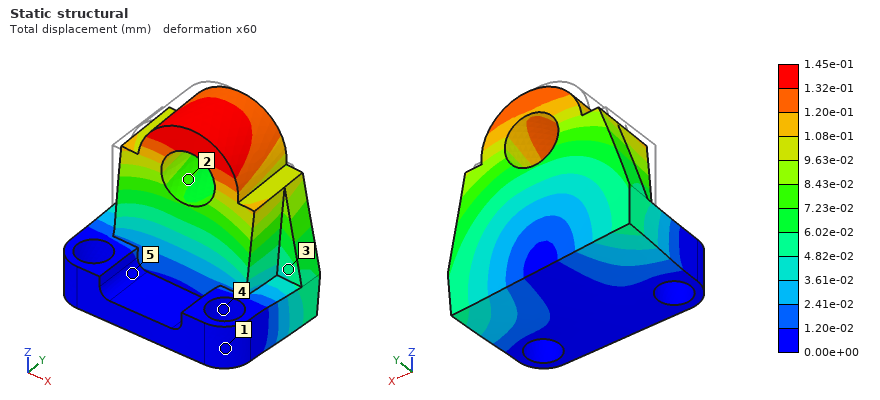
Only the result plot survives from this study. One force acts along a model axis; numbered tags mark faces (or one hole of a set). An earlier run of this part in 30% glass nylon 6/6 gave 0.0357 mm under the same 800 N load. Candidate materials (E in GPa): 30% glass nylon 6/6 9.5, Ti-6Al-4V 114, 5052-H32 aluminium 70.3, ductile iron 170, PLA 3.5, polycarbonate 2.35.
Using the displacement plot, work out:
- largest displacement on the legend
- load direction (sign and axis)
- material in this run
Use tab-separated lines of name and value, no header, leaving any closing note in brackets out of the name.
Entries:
largest displacement on the legend	1.45e-01 mm
load direction	+X
material in this run	polycarbonate
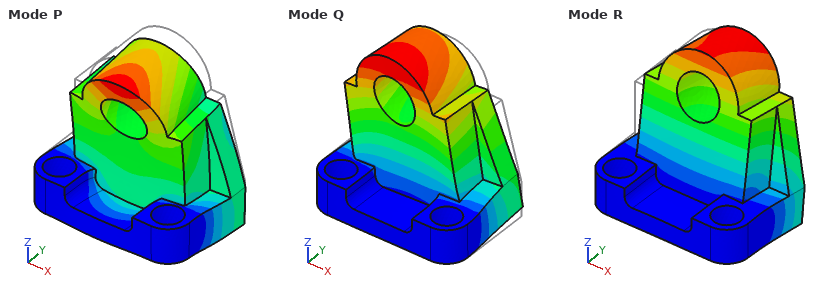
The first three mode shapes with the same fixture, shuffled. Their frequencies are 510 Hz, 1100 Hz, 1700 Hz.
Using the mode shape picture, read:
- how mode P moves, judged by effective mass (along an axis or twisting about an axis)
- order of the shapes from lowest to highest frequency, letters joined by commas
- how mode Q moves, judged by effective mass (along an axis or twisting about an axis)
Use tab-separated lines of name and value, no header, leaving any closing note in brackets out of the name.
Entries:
how mode P moves, judged by effective mass	along Z
order of the shapes from lowest to highest frequency, letters joined by commas	R, Q, P
how mode Q moves, judged by effective mass	along X
